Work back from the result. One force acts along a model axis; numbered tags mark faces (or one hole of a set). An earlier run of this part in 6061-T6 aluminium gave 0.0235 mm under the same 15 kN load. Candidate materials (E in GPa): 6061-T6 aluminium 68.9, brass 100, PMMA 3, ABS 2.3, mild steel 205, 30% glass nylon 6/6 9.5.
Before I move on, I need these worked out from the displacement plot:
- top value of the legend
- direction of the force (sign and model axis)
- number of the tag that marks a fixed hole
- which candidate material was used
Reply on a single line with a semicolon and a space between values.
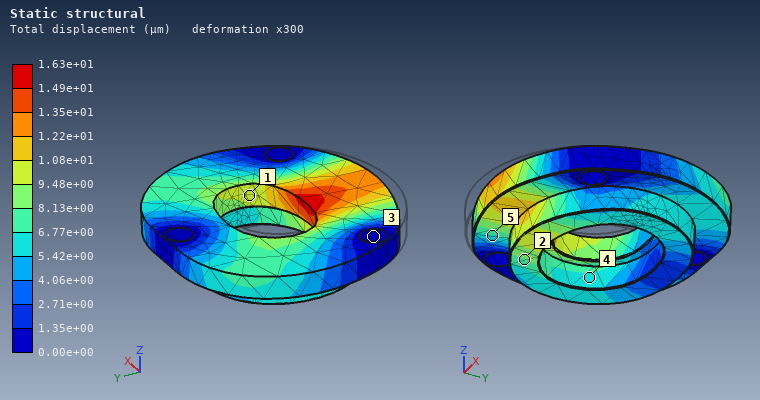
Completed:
1.63e+01 µm; +Y; 3; brass
